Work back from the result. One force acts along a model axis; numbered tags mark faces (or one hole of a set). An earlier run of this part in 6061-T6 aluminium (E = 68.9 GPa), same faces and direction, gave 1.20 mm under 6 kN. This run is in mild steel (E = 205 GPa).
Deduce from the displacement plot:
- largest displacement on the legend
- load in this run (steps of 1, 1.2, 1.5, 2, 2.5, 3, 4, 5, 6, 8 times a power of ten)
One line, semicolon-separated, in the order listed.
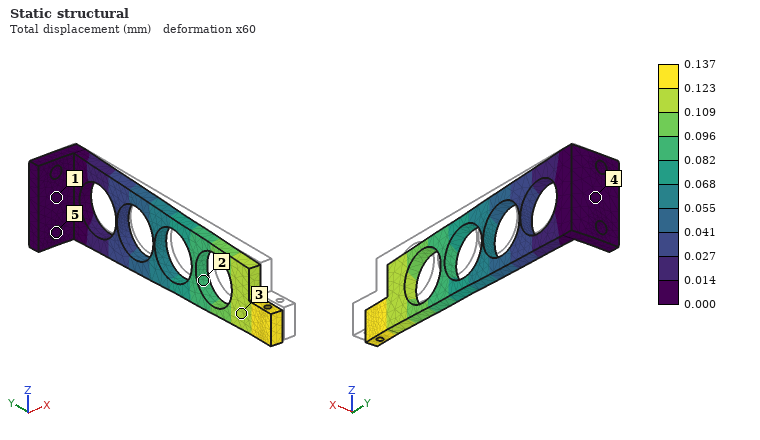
0.137 mm; 2 kN
